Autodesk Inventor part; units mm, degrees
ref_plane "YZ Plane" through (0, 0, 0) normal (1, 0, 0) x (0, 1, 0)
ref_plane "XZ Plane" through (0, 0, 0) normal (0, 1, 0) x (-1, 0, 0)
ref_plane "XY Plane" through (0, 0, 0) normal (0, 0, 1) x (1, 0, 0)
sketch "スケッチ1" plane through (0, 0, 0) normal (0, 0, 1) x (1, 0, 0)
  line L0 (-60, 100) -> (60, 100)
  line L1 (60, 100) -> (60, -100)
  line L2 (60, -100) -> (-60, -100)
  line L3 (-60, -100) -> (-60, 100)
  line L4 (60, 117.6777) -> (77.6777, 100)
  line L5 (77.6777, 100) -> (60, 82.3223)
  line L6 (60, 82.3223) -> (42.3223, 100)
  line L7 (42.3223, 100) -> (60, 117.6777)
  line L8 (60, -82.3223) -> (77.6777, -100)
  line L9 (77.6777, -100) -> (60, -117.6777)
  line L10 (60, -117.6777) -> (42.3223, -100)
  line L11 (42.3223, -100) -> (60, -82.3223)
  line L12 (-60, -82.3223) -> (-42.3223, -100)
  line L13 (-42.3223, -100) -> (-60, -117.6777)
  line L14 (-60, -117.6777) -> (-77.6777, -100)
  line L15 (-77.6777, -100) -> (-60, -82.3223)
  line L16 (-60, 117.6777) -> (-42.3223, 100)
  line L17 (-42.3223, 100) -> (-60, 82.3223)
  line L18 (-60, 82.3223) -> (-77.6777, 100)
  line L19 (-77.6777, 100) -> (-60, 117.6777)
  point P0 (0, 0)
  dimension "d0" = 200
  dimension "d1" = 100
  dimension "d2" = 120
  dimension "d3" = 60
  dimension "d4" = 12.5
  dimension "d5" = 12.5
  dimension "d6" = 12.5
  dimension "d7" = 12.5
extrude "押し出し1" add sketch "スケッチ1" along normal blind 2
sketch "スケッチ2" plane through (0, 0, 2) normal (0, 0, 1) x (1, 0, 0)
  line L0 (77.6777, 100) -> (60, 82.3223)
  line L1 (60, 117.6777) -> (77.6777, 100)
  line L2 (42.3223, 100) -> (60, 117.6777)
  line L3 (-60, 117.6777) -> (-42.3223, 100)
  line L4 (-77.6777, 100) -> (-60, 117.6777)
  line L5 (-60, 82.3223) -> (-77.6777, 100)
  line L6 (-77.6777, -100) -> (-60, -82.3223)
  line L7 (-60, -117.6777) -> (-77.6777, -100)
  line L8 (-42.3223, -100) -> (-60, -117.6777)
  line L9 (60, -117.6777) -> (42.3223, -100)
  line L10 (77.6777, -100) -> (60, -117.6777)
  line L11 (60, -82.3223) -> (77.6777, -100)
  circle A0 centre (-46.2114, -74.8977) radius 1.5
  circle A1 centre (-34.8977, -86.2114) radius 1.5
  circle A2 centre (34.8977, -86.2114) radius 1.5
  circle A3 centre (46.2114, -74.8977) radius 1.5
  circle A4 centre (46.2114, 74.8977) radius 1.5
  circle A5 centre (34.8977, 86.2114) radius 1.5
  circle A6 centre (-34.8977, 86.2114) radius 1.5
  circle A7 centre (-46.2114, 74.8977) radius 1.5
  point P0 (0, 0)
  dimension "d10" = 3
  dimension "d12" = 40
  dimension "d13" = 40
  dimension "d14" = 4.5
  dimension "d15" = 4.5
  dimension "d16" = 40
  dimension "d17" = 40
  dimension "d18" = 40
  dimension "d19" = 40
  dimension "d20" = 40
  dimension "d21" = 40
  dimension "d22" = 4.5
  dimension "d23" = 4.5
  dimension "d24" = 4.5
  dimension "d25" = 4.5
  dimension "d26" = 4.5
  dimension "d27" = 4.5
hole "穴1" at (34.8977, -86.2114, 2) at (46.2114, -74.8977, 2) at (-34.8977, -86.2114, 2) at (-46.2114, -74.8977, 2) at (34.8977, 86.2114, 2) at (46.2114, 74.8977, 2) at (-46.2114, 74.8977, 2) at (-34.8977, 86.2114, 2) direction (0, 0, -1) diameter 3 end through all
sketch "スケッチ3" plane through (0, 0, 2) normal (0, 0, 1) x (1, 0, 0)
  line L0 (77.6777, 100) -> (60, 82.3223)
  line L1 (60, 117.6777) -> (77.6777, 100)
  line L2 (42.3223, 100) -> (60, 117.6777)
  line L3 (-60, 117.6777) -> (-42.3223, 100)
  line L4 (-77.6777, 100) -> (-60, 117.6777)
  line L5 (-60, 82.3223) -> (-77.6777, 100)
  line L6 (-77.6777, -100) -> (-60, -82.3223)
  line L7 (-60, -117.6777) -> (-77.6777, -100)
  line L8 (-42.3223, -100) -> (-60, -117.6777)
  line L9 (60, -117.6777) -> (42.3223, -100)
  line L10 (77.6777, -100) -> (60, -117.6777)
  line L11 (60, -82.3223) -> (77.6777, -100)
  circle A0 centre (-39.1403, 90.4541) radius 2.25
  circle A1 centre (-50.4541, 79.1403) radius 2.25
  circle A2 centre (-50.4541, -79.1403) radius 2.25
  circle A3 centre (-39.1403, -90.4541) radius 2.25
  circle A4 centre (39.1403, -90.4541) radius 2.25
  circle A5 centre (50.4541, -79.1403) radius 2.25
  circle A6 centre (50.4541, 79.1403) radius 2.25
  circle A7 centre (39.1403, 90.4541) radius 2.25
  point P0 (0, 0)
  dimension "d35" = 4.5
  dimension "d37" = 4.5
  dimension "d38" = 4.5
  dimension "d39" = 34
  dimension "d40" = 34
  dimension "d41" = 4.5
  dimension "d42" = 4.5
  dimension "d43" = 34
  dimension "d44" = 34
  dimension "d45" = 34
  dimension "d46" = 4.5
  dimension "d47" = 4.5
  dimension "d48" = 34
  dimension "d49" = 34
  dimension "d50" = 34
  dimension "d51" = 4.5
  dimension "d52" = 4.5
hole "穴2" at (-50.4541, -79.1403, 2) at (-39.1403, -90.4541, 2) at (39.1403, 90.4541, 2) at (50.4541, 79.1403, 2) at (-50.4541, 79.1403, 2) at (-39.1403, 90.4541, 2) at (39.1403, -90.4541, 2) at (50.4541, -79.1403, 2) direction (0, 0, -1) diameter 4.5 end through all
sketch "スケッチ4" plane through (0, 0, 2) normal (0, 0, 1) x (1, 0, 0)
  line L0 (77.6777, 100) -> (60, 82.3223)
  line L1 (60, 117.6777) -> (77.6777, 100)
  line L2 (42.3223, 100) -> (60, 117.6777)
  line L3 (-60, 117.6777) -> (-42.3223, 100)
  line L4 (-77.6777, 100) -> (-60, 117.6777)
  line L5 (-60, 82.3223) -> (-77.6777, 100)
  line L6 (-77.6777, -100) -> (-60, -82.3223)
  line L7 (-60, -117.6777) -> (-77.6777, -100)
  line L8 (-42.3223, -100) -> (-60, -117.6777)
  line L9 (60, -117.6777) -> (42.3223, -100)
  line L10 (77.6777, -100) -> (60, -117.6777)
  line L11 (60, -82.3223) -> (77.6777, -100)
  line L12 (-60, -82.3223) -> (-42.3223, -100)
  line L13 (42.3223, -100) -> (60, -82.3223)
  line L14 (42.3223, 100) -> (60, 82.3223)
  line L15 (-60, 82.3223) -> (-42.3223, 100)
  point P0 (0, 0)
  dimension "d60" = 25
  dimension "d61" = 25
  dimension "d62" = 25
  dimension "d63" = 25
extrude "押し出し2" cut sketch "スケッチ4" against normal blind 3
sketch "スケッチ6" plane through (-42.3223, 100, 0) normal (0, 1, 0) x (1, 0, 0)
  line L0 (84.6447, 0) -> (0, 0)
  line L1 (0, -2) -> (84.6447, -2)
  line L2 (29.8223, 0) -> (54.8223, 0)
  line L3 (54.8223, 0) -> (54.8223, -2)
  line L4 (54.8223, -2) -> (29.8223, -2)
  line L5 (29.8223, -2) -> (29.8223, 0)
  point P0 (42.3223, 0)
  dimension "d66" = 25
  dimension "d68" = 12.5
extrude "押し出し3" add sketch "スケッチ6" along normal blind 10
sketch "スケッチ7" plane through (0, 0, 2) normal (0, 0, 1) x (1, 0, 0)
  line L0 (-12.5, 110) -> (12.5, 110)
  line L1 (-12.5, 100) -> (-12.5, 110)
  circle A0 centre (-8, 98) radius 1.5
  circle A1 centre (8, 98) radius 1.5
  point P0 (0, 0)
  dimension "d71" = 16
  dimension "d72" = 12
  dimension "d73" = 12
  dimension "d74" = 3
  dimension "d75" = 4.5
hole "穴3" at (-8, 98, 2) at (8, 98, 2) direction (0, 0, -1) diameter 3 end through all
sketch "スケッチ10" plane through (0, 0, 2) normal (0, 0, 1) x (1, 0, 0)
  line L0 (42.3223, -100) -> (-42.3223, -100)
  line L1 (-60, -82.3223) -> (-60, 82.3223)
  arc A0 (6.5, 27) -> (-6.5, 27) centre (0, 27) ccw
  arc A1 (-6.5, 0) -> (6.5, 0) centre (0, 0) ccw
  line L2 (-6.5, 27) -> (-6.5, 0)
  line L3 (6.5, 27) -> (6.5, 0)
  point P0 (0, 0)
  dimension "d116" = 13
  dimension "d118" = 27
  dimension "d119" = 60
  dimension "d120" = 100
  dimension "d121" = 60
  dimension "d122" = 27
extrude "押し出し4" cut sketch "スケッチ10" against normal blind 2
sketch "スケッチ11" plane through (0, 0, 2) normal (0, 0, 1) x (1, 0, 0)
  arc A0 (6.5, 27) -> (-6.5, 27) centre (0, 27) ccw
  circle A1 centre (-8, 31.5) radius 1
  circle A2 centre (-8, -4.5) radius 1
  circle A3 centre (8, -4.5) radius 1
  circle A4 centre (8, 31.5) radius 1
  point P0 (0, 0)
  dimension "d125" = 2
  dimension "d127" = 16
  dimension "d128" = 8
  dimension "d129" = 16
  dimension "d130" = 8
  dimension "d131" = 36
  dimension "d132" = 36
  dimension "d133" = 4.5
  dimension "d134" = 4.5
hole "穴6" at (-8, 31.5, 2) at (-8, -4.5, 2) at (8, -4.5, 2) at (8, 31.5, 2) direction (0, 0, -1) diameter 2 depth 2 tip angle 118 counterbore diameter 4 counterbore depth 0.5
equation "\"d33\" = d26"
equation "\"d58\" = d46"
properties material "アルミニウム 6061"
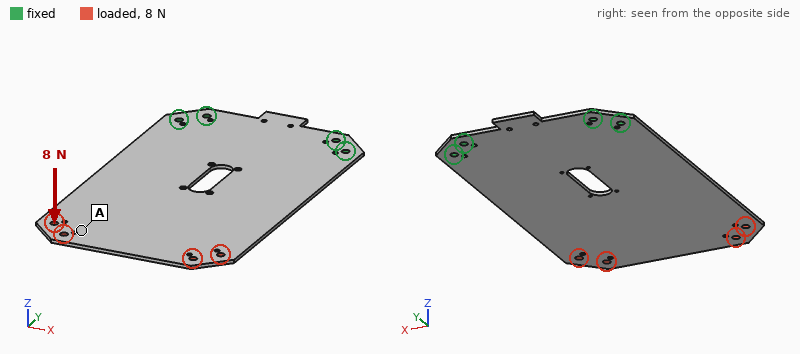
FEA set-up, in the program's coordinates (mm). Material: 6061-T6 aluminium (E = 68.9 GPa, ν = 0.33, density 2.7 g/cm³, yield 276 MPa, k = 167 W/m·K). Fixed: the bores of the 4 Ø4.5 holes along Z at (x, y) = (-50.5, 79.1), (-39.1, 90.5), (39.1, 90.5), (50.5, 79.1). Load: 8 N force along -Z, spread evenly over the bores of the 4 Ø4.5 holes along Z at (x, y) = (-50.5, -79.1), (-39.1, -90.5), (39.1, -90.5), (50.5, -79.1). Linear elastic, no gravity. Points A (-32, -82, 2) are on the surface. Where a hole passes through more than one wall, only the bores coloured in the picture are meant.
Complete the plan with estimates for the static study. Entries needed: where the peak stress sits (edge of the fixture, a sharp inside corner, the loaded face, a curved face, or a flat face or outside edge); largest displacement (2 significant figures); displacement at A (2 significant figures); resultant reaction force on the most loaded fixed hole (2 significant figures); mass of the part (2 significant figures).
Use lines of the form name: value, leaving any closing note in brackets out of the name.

where the peak stress sits: a curved face
largest displacement: 2.8 mm
displacement at A: 2.4 mm
resultant reaction force on the most loaded fixed hole: 17 N
mass of the part: 120 g
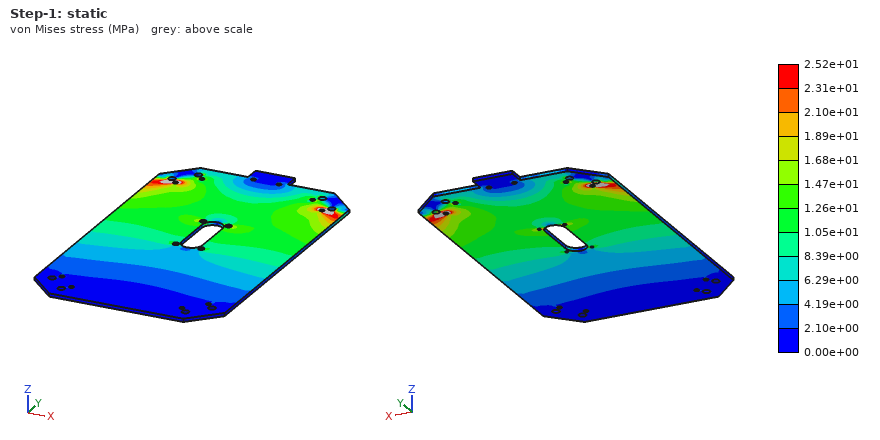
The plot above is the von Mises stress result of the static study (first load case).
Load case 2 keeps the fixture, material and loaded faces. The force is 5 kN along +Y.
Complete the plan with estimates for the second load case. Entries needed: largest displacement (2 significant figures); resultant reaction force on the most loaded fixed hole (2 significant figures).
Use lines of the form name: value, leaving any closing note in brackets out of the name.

largest displacement: 76 µm
resultant reaction force on the most loaded fixed hole: 1.3 kN
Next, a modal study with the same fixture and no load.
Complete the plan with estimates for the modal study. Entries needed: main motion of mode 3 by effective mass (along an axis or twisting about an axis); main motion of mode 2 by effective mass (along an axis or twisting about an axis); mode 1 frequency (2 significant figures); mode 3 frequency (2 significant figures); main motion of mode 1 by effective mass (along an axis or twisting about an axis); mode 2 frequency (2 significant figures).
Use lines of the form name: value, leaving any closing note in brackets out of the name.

main motion of mode 3 by effective mass: along Z
main motion of mode 2 by effective mass: twisting about Y
mode 1 frequency: 48 Hz
mode 3 frequency: 310 Hz
main motion of mode 1 by effective mass: along Z
mode 2 frequency: 180 Hz
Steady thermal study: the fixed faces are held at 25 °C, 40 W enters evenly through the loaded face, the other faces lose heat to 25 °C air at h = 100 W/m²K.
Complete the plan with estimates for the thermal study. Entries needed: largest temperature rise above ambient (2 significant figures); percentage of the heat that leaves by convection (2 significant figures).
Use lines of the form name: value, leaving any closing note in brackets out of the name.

largest temperature rise above ambient: 44 K
percentage of the heat that leaves by convection: 98 %
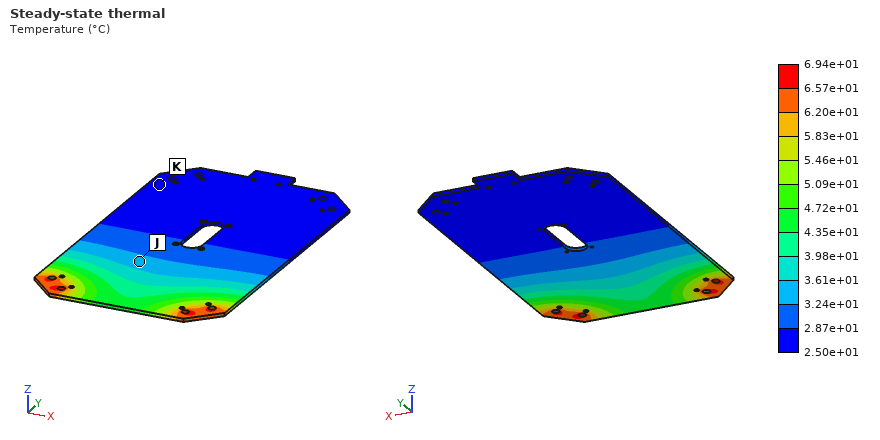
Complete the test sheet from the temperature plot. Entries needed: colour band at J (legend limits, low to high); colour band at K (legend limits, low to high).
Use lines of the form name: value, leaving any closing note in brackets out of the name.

colour band at J: 3.24e+01 to 3.61e+01 °C
colour band at K: 2.50e+01 to 2.87e+01 °C
